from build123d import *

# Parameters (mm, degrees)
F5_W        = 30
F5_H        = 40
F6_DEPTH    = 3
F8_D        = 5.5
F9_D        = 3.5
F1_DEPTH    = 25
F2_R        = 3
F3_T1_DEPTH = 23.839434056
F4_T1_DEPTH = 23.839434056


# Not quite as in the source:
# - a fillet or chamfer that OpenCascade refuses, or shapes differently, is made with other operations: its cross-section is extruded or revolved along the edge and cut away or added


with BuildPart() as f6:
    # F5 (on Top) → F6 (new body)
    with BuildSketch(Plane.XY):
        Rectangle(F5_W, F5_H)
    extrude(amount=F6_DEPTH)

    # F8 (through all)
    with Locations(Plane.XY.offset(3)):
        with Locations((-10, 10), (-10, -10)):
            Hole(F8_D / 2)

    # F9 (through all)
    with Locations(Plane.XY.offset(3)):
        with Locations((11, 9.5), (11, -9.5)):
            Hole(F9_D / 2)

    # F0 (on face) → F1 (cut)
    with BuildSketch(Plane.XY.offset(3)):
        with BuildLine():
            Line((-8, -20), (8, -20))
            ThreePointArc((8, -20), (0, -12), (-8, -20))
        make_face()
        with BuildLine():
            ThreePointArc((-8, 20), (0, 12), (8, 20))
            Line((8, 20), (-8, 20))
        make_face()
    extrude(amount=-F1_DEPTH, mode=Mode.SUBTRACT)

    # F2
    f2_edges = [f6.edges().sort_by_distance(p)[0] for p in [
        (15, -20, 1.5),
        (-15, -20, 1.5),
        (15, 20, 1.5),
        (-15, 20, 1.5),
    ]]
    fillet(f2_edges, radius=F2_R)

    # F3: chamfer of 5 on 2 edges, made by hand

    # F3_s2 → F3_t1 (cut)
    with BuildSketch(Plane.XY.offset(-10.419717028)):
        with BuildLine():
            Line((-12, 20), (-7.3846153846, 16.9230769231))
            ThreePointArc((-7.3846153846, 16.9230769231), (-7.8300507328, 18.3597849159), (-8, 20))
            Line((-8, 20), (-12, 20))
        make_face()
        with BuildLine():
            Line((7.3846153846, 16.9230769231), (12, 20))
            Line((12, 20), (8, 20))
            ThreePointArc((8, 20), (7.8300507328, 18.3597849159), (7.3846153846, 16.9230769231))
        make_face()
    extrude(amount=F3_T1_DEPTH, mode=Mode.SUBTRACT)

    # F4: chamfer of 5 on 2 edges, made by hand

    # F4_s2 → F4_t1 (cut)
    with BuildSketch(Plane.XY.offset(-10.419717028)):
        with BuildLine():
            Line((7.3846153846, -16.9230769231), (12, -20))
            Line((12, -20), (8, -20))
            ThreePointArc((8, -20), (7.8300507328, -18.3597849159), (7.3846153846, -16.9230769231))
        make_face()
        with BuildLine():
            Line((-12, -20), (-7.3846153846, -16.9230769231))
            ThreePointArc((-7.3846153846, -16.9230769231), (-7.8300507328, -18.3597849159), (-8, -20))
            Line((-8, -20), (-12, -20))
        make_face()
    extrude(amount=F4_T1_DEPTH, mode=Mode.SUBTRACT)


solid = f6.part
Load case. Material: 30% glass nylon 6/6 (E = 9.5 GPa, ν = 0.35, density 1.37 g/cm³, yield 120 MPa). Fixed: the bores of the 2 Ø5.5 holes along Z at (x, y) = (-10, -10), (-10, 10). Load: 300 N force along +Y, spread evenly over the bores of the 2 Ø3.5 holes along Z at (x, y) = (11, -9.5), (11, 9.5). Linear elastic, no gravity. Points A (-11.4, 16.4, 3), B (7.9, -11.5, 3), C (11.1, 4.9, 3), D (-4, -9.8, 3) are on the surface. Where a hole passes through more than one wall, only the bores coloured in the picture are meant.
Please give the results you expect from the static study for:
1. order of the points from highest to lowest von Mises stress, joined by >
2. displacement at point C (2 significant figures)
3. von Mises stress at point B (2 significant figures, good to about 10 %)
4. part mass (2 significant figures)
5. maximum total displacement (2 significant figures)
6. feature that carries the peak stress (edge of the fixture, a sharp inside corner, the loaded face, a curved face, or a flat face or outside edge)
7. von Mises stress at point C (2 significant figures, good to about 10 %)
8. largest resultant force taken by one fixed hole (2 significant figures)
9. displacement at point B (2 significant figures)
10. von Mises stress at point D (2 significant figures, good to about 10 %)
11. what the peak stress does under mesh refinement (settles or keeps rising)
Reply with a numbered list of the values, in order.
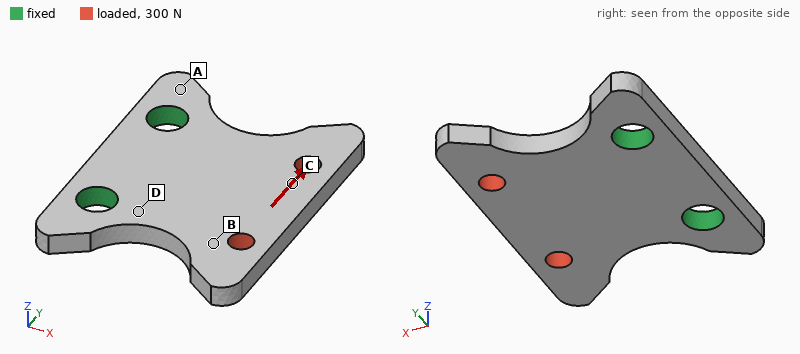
1. D > C > B > A
2. 39 µm
3. 3.8 MPa
4. 3.7 g
5. 60 µm
6. edge of the fixture
7. 6.3 MPa
8. 310 N
9. 37 µm
10. 12 MPa
11. keeps rising
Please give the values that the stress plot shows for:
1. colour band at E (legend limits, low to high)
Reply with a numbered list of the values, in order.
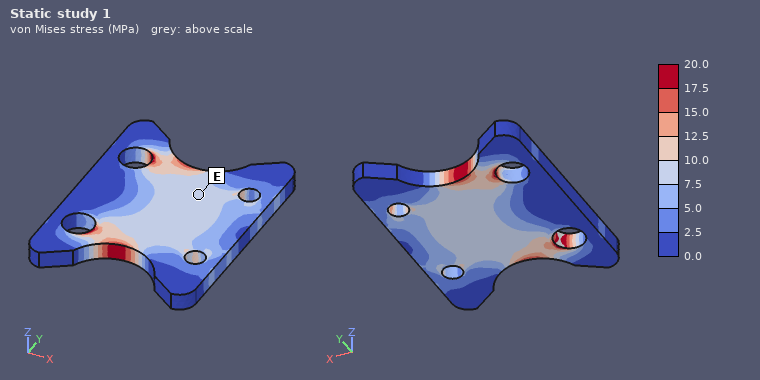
1. 7.5 to 10.0 MPa
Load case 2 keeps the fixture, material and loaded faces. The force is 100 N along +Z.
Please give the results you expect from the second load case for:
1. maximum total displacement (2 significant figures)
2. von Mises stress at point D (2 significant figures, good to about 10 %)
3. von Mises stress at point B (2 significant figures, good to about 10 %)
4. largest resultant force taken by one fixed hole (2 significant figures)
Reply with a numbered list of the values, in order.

1. 0.58 mm
2. 43 MPa
3. 7.2 MPa
4. 50 N
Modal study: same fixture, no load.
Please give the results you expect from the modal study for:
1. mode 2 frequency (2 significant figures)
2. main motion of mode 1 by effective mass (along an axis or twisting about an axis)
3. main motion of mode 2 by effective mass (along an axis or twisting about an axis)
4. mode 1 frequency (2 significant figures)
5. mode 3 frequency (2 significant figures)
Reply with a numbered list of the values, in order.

1. 3300 Hz
2. along Z
3. twisting about X
4. 2000 Hz
5. 7200 Hz
